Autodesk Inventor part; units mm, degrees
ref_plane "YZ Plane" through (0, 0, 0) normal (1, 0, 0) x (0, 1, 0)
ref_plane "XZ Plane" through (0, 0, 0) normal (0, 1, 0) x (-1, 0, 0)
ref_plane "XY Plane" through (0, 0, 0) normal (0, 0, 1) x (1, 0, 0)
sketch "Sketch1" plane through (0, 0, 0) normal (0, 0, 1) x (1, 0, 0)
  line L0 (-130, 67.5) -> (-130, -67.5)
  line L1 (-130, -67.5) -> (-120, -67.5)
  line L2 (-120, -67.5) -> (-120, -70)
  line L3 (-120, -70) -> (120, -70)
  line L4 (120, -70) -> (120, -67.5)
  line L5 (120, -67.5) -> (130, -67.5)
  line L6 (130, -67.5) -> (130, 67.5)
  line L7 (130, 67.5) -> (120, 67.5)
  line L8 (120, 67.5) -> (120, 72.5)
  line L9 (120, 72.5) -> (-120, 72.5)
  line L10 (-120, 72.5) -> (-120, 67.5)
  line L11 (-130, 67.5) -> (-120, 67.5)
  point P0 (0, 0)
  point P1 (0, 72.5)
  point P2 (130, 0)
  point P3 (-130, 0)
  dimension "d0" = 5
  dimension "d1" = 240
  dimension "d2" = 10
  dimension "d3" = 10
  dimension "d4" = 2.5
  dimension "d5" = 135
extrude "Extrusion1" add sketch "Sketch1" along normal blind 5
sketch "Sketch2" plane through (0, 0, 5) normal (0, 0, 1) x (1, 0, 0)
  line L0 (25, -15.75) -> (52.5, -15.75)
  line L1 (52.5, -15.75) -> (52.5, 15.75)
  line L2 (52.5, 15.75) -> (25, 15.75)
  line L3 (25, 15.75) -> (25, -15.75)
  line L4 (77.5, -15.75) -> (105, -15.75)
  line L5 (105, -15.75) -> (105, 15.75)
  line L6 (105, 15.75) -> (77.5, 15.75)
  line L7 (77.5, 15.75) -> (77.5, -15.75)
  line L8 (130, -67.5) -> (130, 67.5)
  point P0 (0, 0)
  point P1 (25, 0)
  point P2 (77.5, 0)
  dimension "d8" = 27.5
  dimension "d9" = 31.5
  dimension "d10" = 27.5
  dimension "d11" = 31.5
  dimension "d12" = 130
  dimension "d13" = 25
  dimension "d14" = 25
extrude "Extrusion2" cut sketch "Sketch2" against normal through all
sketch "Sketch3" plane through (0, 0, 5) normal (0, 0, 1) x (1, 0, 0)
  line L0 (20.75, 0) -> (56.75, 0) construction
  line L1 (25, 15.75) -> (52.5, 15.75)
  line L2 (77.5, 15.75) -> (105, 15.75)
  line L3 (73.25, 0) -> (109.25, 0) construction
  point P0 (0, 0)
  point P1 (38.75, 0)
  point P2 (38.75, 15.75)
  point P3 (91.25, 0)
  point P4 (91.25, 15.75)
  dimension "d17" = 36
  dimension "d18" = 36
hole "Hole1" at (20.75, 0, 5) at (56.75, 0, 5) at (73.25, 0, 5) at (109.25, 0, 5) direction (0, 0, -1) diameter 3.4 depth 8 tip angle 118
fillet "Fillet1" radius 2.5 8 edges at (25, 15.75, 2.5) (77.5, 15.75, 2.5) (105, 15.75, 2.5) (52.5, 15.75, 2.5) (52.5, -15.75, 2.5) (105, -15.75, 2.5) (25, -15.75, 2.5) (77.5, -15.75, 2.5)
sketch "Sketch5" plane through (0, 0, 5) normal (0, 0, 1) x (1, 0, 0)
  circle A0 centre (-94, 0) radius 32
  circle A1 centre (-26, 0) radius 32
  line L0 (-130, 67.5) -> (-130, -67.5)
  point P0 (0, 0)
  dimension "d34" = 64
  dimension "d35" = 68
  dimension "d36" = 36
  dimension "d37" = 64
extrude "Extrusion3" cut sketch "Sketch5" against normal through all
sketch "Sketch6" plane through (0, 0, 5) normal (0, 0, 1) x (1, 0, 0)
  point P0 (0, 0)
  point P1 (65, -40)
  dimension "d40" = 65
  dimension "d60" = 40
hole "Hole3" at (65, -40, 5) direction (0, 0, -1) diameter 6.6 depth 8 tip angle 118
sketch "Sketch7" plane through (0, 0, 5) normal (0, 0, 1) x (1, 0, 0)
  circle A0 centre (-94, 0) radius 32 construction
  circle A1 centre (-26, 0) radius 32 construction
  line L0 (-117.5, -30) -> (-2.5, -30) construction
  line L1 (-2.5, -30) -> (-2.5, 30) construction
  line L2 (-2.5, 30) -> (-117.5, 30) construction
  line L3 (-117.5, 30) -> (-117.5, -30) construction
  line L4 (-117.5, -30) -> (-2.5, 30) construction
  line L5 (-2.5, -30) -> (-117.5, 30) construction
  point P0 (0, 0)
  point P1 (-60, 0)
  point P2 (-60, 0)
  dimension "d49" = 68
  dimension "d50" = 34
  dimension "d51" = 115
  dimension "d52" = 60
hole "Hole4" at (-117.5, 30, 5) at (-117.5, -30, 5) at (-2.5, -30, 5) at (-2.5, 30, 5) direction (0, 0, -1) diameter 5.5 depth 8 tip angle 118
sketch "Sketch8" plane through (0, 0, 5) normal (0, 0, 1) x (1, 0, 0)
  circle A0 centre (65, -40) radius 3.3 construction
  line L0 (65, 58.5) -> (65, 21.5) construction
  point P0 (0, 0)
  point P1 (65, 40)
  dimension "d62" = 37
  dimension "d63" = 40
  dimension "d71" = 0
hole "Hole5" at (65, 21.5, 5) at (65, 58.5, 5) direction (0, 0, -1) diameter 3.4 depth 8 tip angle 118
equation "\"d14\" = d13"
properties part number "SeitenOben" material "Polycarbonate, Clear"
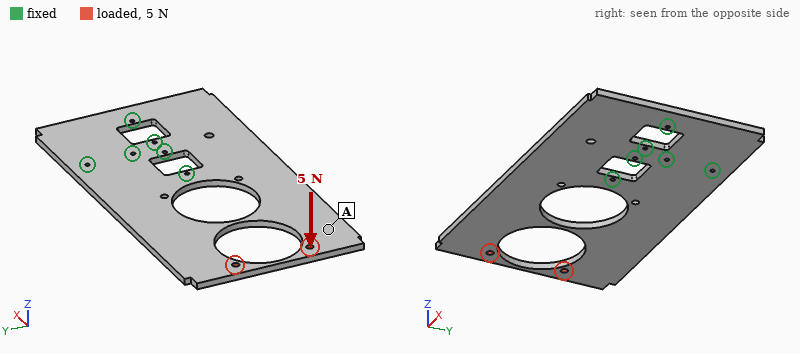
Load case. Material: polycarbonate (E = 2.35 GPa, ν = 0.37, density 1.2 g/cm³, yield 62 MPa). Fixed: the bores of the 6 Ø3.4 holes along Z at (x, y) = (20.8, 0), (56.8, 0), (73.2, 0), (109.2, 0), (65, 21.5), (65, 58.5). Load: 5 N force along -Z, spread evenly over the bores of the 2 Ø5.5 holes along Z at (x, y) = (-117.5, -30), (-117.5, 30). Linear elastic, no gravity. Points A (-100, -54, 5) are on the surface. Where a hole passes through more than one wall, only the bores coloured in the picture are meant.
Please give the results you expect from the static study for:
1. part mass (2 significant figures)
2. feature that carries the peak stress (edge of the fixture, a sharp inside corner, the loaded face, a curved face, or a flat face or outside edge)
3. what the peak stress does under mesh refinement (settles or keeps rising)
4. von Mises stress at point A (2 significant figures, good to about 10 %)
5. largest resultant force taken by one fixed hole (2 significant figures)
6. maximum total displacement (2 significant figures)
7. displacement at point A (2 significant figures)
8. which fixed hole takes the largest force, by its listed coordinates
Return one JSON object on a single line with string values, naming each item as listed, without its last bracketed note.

{"part mass": "170 g", "feature that carries the peak stress": "edge of the fixture", "what the peak stress does under mesh refinement": "keeps rising", "von Mises stress at point A": "0.32 MPa", "largest resultant force taken by one fixed hole": "14 N", "maximum total displacement": "3.0 mm", "displacement at point A": "2.2 mm", "which fixed hole takes the largest force, by its listed coordinates": "(20.8, 0)"}
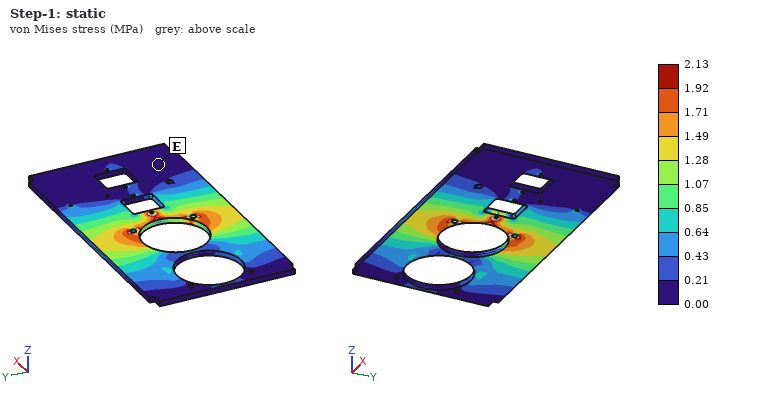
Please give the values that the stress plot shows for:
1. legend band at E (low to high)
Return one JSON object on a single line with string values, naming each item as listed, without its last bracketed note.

{"legend band at E": "0.00 to 0.21 MPa"}
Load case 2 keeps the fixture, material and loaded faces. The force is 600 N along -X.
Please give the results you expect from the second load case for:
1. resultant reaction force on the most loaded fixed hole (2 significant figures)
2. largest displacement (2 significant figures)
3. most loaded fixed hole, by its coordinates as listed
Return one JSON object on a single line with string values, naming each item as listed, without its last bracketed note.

{"resultant reaction force on the most loaded fixed hole": "150 N", "largest displacement": "0.25 mm", "most loaded fixed hole, by its coordinates as listed": "(20.8, 0)"}
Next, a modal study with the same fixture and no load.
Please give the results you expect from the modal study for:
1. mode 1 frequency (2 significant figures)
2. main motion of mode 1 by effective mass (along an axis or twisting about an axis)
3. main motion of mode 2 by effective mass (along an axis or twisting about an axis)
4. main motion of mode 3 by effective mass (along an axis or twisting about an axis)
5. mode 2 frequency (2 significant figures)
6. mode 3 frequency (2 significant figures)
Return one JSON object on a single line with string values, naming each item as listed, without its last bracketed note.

{"mode 1 frequency": "40 Hz", "main motion of mode 1 by effective mass": "along Z", "main motion of mode 2 by effective mass": "twisting about X", "main motion of mode 3 by effective mass": "along Z", "mode 2 frequency": "75 Hz", "mode 3 frequency": "170 Hz"}
